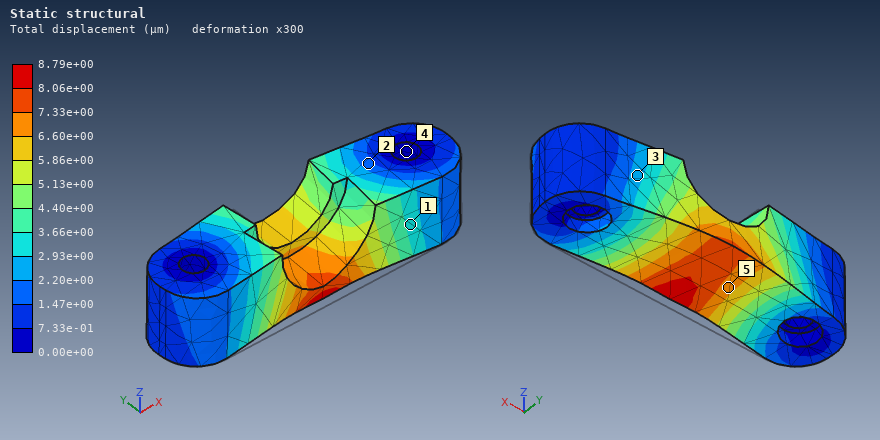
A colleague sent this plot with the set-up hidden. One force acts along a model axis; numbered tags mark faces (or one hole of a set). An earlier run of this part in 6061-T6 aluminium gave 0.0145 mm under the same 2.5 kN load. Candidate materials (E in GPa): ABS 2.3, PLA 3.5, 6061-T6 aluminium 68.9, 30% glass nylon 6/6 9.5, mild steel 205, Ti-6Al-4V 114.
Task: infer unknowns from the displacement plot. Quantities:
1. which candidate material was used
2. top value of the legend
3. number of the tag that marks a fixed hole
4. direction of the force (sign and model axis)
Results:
Ti-6Al-4V
8.79e+00 µm
4
+Y
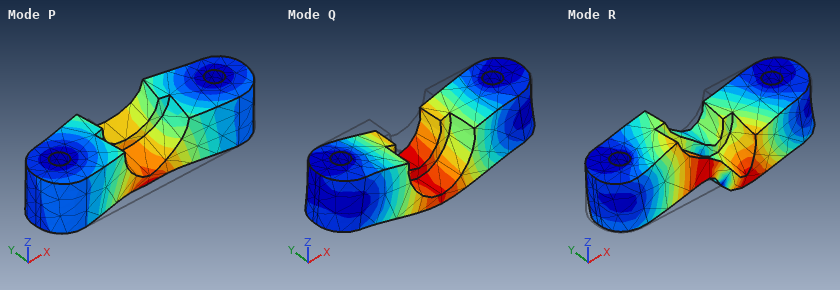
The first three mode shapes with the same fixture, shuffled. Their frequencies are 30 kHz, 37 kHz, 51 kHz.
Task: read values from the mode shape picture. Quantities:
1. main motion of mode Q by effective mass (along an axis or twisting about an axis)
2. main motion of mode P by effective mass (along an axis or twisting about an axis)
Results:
along Z
along Y
